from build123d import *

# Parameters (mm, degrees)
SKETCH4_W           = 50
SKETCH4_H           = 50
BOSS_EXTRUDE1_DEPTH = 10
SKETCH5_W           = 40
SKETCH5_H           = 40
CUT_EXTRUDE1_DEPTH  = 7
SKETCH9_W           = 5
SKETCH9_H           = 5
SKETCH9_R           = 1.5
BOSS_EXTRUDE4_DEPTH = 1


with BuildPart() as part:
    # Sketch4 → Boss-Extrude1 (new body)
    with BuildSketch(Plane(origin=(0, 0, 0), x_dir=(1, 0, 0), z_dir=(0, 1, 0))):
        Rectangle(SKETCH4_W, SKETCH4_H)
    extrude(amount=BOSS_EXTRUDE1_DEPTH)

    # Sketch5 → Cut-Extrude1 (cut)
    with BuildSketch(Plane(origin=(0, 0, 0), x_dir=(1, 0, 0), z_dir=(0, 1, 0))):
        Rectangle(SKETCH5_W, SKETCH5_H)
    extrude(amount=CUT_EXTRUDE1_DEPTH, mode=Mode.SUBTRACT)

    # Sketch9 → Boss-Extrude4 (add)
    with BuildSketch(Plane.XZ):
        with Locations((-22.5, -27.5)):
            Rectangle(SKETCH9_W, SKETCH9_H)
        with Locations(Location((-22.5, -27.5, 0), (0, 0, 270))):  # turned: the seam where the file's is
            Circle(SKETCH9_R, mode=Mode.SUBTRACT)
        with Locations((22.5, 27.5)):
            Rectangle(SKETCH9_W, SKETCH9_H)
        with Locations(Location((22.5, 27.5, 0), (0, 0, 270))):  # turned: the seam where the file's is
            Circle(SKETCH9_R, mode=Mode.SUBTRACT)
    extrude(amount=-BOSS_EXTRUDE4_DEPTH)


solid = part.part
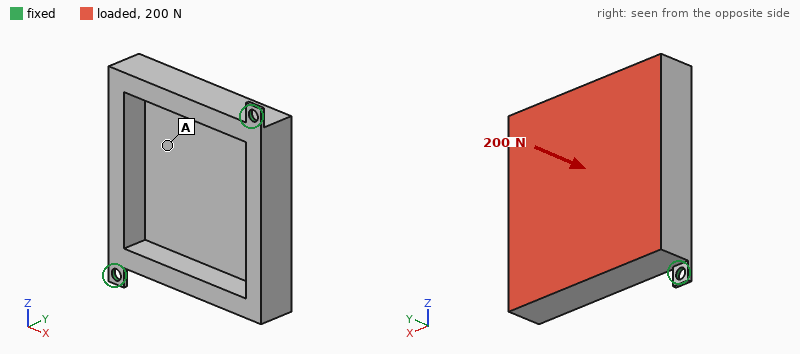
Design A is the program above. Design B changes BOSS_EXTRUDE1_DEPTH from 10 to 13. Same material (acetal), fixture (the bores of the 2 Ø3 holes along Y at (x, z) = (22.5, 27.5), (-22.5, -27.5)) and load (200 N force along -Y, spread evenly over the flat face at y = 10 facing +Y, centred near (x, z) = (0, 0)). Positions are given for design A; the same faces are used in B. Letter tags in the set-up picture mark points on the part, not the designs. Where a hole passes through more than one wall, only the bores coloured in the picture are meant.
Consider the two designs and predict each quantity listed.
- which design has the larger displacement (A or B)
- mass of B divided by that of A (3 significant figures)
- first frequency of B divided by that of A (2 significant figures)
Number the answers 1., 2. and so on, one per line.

1. A
2. 1.54
3. 0.79
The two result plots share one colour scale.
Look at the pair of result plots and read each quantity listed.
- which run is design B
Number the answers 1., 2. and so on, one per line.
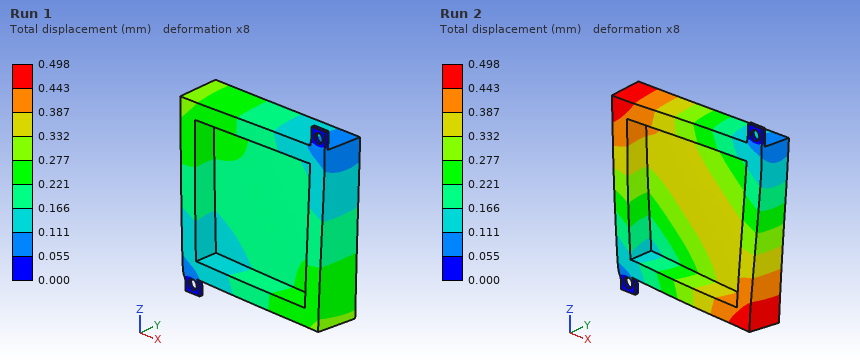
1. Run 1
